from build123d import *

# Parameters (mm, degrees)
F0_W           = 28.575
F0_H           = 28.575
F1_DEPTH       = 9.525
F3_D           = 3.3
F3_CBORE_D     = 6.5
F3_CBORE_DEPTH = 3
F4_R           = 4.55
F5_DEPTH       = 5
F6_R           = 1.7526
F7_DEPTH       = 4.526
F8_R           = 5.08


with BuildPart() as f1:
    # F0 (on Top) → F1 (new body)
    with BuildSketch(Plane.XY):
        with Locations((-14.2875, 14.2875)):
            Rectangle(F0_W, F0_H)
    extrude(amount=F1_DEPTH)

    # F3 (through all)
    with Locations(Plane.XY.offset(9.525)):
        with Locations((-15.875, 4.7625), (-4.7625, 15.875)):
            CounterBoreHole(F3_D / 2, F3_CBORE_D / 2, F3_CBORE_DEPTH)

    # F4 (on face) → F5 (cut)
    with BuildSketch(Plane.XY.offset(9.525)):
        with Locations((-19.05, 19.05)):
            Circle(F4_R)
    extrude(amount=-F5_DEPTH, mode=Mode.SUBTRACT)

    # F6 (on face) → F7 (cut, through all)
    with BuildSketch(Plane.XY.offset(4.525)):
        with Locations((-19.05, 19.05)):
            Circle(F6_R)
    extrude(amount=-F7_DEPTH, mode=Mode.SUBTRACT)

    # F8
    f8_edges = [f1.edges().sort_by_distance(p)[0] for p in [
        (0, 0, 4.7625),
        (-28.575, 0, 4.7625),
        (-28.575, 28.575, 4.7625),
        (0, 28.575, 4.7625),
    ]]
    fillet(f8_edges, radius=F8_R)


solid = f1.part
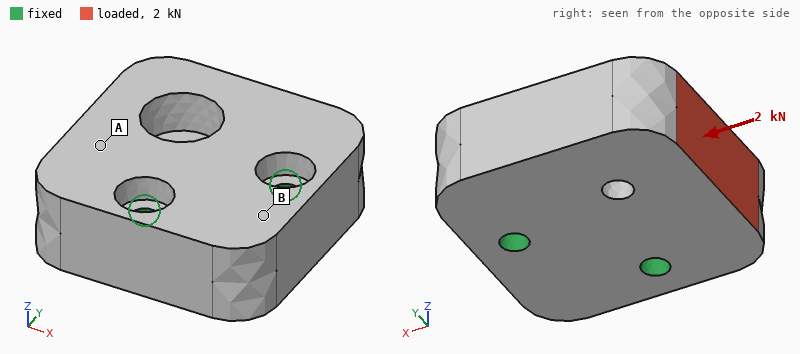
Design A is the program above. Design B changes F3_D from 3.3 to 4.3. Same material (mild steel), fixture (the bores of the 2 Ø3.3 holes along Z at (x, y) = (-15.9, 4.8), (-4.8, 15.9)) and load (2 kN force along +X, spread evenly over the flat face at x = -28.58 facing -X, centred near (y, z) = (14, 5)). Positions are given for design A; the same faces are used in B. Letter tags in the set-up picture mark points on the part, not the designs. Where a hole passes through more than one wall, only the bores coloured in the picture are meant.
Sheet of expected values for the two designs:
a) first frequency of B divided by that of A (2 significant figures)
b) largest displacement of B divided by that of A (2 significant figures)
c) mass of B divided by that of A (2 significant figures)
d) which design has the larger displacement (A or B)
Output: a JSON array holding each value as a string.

["1.1", "0.91", "0.99", "A"]
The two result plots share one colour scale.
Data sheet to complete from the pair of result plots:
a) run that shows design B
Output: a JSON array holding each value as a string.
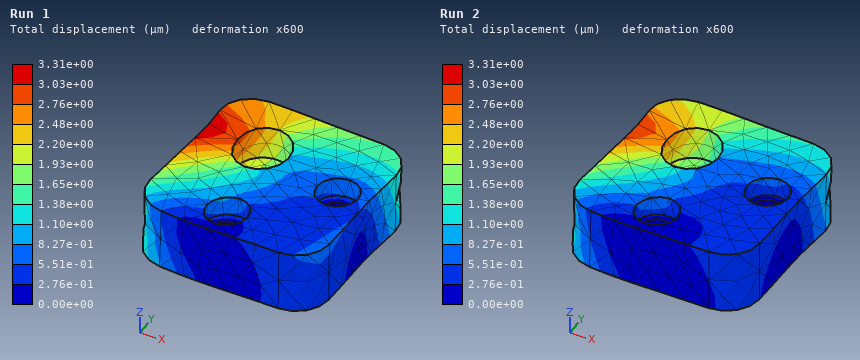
["Run 2"]
